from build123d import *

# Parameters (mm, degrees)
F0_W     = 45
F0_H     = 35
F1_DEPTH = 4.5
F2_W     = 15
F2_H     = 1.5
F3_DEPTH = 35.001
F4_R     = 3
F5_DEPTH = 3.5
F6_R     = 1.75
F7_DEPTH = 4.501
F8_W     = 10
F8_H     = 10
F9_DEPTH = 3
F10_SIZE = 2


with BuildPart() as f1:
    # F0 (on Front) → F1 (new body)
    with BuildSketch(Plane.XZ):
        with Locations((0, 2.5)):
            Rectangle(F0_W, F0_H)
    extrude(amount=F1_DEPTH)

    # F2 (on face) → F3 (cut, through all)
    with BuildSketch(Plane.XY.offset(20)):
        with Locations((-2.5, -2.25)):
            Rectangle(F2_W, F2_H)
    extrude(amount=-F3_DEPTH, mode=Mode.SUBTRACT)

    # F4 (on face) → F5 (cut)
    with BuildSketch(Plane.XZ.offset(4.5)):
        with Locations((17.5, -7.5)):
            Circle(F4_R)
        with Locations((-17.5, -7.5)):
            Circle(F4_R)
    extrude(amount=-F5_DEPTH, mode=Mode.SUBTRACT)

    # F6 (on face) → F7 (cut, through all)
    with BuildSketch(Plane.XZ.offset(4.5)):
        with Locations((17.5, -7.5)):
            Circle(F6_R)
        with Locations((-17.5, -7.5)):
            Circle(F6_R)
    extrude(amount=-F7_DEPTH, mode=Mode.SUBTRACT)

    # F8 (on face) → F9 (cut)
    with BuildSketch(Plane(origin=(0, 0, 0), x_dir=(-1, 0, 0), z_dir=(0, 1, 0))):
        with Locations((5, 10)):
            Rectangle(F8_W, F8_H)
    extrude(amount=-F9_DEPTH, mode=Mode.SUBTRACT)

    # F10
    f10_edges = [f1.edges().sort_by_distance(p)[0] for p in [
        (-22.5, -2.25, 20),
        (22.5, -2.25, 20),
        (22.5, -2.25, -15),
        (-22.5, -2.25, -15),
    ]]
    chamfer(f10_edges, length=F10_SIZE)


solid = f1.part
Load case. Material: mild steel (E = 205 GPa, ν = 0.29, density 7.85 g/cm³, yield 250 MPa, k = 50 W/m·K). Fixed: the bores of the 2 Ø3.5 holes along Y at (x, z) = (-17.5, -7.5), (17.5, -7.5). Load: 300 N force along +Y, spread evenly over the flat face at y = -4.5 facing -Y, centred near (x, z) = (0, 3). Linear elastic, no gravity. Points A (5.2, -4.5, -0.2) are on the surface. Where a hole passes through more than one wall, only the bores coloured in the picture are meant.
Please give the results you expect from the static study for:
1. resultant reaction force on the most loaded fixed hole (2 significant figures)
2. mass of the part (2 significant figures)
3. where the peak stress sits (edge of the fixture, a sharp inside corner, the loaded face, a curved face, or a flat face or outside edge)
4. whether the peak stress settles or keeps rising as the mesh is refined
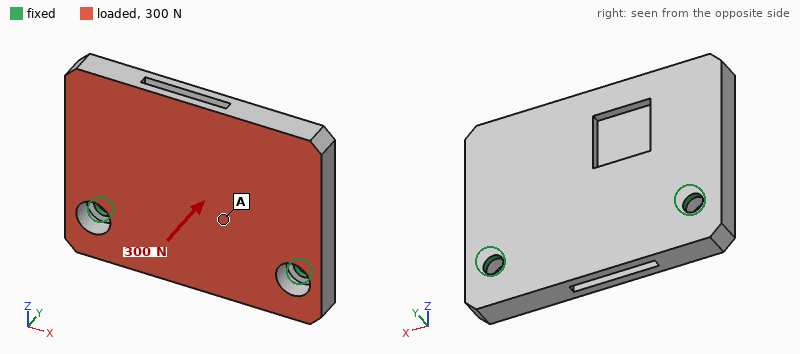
190 N
46 g
edge of the fixture
keeps rising
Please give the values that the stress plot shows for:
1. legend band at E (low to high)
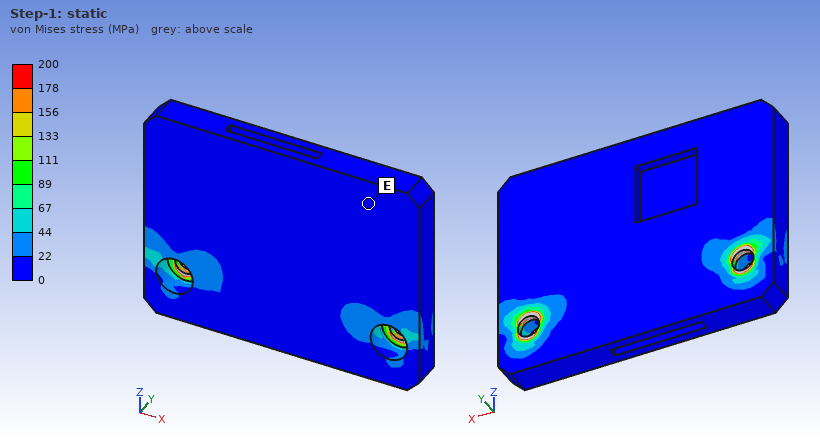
0 to 22 MPa
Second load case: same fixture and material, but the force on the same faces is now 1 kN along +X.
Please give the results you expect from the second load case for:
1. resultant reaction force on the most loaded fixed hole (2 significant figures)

590 N
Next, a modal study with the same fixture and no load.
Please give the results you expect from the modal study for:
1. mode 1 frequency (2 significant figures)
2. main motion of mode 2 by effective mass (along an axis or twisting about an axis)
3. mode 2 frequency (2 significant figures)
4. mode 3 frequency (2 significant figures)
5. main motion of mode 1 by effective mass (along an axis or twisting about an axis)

2000 Hz
twisting about Z
5100 Hz
11 kHz
along Y
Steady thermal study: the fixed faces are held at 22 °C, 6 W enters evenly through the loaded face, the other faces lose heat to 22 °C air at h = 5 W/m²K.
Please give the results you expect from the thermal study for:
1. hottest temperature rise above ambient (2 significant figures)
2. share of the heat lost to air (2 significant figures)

17 K
3.4 %
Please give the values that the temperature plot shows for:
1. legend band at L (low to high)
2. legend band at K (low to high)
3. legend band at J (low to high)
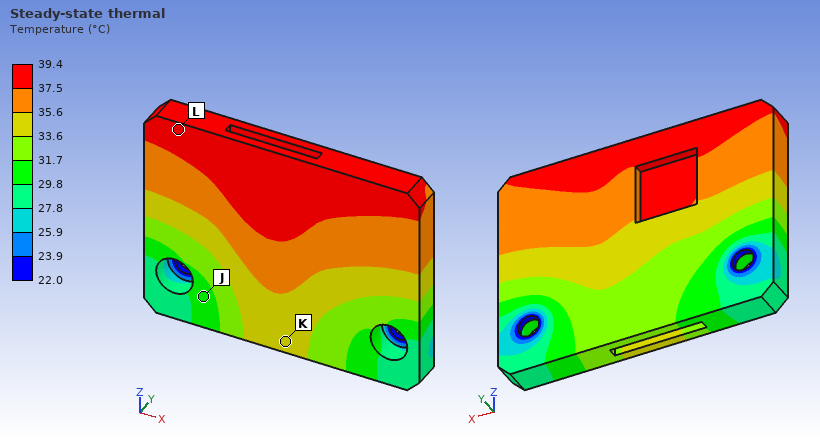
37.5 to 39.4 °C
33.6 to 35.6 °C
29.8 to 31.7 °C
